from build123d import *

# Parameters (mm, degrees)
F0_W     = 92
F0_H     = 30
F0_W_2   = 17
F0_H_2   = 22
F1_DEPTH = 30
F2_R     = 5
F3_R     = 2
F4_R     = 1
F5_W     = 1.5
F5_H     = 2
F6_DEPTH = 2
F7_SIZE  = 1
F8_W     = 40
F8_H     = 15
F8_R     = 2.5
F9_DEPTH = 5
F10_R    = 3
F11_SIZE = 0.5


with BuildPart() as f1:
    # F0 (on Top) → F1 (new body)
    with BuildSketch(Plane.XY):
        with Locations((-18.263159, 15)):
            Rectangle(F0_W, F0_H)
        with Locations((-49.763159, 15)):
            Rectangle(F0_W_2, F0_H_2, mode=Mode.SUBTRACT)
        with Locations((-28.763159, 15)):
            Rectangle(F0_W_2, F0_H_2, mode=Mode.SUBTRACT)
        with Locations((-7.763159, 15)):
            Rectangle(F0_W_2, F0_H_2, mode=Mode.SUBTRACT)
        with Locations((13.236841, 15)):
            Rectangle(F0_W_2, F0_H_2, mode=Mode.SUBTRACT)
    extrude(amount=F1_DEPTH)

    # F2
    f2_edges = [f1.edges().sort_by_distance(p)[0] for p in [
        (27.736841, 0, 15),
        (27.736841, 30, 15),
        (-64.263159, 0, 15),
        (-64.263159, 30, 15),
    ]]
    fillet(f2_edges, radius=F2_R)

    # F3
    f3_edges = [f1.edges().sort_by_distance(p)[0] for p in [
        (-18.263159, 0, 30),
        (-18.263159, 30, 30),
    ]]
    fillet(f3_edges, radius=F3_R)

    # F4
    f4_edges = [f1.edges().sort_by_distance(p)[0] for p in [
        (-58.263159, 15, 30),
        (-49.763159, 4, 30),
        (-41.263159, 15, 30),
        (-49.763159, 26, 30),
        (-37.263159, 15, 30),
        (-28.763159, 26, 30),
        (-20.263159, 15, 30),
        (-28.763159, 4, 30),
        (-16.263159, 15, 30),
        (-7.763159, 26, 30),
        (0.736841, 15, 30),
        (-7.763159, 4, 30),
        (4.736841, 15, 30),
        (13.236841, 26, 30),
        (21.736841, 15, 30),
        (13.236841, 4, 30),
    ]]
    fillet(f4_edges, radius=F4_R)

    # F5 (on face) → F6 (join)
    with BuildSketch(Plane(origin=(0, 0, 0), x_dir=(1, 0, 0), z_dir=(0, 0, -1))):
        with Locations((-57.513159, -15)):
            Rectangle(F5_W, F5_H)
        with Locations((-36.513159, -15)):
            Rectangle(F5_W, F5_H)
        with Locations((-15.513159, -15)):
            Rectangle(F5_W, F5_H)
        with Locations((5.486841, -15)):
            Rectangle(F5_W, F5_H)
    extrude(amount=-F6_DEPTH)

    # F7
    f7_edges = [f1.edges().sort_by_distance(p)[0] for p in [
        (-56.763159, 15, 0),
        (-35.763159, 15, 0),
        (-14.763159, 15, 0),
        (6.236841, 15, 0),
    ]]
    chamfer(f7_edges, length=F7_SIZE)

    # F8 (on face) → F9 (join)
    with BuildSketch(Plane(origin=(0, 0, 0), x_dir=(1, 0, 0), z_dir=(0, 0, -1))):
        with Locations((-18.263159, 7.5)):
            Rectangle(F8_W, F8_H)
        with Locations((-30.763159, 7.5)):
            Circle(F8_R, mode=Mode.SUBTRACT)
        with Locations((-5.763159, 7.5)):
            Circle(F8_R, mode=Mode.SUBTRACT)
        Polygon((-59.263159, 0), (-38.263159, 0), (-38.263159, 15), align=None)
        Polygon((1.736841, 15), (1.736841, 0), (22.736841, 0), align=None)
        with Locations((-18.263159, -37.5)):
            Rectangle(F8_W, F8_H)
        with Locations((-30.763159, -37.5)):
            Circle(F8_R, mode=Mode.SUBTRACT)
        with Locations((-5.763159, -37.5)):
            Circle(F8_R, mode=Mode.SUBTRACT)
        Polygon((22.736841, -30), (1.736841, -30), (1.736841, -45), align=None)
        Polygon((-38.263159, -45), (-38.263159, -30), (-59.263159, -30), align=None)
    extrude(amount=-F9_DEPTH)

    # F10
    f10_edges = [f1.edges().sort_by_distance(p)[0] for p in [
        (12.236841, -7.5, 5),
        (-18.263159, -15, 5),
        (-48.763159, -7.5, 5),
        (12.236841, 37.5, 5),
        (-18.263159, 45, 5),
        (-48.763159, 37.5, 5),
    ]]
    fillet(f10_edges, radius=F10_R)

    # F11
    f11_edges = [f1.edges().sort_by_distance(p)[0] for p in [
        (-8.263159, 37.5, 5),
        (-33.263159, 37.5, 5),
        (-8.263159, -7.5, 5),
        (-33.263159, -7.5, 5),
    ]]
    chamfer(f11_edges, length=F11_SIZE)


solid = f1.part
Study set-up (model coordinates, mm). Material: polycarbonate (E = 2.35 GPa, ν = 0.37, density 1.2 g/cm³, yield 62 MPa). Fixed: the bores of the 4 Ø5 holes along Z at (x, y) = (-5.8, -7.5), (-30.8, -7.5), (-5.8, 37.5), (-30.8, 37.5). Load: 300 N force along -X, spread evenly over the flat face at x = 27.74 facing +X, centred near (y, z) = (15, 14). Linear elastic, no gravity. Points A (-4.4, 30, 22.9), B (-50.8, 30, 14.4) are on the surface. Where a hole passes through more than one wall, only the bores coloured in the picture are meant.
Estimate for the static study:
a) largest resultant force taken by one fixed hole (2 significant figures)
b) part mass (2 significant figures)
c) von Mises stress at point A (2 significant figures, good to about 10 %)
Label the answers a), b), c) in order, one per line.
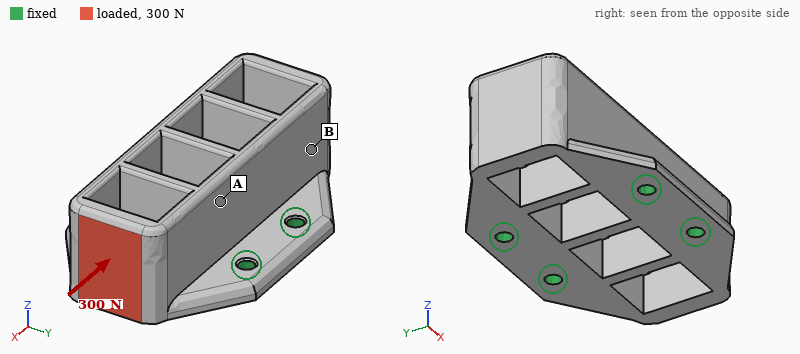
a) 110 N
b) 55 g
c) 1.5 MPa
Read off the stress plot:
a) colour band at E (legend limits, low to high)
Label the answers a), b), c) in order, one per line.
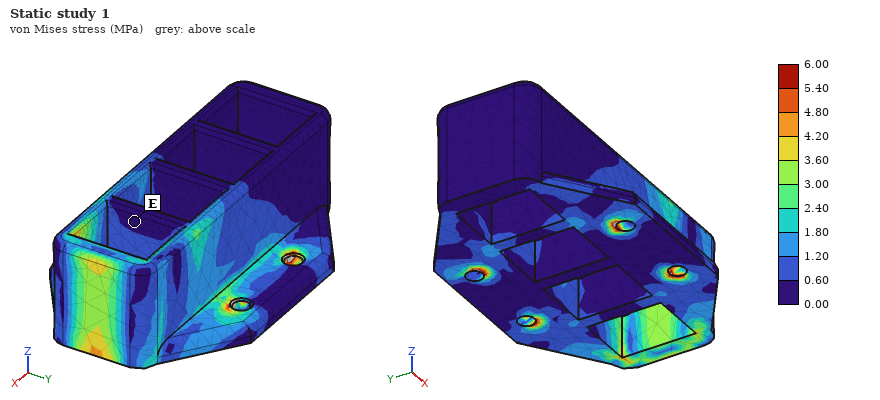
a) 0.00 to 0.60 MPa
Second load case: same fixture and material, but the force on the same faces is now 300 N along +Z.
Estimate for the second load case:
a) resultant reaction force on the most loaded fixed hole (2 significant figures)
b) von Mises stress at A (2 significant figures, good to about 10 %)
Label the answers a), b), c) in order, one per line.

a) 340 N
b) 2.8 MPa
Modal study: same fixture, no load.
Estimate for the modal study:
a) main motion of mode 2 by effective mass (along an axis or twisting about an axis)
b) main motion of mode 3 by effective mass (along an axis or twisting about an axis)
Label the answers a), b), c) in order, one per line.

a) twisting about Z
b) along Y
